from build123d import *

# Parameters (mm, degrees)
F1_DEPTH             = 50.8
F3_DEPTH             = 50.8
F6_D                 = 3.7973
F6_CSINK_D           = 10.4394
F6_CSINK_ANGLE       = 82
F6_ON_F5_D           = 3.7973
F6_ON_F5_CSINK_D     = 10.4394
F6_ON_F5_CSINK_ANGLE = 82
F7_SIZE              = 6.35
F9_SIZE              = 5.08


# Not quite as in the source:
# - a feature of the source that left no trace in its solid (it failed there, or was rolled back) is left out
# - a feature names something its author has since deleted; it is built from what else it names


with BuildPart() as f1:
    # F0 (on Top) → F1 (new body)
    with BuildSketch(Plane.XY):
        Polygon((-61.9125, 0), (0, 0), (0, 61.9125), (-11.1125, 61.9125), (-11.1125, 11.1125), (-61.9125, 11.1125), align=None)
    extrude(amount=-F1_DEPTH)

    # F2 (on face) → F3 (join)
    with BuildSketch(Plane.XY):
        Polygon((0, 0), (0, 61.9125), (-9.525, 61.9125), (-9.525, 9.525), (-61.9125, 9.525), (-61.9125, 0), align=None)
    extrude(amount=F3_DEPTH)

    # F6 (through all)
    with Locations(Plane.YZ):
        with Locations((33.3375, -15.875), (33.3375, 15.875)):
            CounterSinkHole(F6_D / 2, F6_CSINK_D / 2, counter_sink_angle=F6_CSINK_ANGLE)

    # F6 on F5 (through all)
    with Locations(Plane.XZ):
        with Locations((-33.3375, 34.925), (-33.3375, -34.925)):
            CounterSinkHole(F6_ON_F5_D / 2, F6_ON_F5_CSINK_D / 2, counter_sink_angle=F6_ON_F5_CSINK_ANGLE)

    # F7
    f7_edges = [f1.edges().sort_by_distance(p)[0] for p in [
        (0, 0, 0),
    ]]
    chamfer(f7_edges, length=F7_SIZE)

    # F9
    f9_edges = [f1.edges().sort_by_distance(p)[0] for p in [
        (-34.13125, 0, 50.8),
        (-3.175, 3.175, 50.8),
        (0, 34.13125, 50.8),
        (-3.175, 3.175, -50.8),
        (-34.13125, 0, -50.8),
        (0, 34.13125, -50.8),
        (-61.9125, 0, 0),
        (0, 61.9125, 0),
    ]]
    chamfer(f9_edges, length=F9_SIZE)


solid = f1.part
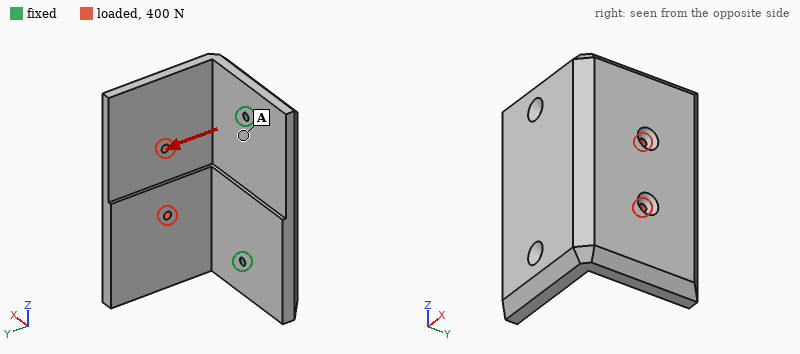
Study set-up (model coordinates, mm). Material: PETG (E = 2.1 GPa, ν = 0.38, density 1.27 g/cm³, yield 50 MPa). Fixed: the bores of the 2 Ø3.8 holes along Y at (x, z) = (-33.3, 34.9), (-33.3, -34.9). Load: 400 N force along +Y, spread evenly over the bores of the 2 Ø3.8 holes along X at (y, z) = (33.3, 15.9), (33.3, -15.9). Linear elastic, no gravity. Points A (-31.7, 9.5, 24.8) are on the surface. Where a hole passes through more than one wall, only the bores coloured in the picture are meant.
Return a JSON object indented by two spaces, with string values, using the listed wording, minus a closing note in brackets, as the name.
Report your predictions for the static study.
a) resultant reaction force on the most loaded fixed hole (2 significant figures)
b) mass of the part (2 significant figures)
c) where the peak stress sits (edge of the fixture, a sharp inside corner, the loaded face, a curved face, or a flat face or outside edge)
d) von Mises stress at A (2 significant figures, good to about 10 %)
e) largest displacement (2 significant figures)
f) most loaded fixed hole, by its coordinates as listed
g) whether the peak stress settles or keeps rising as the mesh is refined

{
  "resultant reaction force on the most loaded fixed hole": "220 N",
  "mass of the part": "140 g",
  "where the peak stress sits": "edge of the fixture",
  "von Mises stress at A": "3.5 MPa",
  "largest displacement": "1.4 mm",
  "most loaded fixed hole, by its coordinates as listed": "(-33.3, -34.9)",
  "whether the peak stress settles or keeps rising as the mesh is refined": "keeps rising"
}
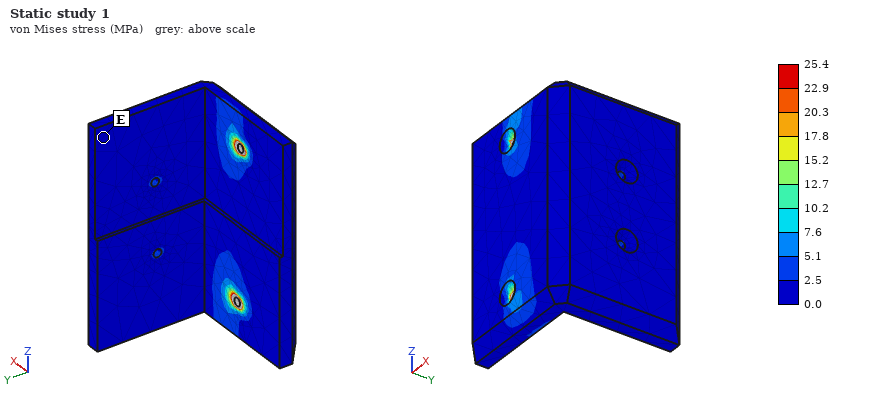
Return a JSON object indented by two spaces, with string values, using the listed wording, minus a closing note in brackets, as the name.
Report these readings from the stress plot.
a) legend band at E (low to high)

{
  "legend band at E": "0.0 to 2.5 MPa"
}
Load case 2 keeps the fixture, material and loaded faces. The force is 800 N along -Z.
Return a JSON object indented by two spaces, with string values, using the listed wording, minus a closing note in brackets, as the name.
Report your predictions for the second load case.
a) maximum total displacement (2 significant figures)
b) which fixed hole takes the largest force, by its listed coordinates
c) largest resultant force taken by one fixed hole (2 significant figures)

{
  "maximum total displacement": "0.93 mm",
  "which fixed hole takes the largest force, by its listed coordinates": "(-33.3, -34.9)",
  "largest resultant force taken by one fixed hole": "630 N"
}
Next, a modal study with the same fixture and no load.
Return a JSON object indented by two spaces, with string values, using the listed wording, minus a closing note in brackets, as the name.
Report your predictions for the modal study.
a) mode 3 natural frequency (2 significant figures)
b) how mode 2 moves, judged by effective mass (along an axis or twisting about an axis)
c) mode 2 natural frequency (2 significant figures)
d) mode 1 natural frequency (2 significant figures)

{
  "mode 3 natural frequency": "860 Hz",
  "how mode 2 moves, judged by effective mass": "along Z",
  "mode 2 natural frequency": "600 Hz",
  "mode 1 natural frequency": "270 Hz"
}
